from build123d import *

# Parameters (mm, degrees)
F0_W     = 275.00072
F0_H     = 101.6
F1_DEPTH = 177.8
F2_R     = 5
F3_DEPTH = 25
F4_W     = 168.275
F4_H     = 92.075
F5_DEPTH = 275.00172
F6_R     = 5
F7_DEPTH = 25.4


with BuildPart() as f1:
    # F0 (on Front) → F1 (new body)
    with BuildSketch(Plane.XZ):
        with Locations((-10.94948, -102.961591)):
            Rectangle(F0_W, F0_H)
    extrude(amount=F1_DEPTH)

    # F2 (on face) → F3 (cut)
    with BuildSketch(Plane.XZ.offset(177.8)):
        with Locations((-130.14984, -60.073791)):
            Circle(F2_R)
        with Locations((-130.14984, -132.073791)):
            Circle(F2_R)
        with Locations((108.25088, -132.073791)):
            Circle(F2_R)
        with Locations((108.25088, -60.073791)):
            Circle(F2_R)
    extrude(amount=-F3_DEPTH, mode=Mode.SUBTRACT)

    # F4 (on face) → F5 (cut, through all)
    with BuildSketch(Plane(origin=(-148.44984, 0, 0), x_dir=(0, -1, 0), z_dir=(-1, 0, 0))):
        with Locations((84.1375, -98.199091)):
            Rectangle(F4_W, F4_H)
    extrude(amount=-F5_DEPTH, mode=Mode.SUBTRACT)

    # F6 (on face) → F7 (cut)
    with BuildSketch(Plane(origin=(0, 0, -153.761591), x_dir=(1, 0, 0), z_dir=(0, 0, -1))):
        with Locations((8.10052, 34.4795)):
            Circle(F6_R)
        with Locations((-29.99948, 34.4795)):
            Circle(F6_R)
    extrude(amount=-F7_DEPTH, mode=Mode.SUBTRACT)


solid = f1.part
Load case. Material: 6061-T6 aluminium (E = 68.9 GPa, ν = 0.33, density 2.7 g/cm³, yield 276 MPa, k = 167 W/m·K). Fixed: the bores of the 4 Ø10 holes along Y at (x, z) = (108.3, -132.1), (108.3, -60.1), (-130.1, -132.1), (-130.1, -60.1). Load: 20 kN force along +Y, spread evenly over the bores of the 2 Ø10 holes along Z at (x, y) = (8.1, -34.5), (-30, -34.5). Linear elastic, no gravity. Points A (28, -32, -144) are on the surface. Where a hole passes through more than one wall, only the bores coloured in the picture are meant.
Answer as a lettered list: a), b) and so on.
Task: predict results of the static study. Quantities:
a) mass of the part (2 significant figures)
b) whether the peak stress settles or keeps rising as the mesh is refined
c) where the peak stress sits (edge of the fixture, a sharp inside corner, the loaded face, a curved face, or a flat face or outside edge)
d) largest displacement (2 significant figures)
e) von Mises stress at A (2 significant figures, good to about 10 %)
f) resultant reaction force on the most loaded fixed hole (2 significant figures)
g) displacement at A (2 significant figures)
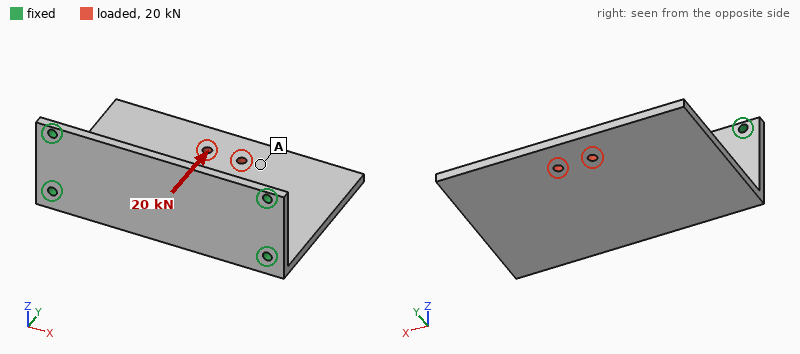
a) 1.9 kg
b) keeps rising
c) edge of the fixture
d) 0.64 mm
e) 14 MPa
f) 12 kN
g) 0.50 mm
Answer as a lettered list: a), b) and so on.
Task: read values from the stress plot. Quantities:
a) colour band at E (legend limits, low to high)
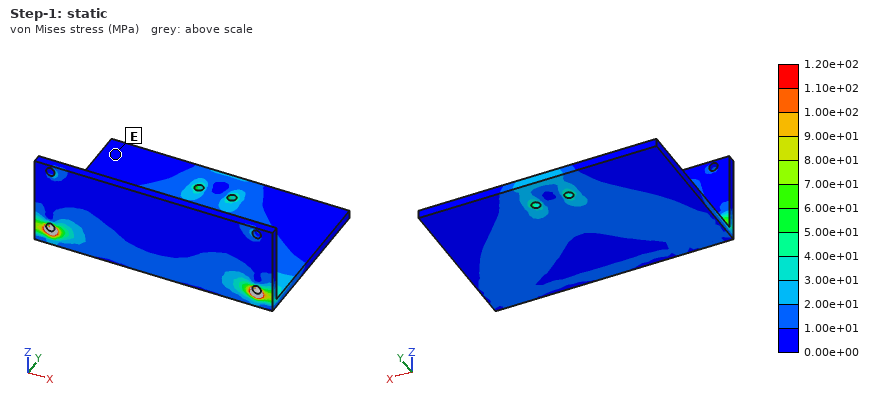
a) 0.00e+00 to 1.00e+01 MPa
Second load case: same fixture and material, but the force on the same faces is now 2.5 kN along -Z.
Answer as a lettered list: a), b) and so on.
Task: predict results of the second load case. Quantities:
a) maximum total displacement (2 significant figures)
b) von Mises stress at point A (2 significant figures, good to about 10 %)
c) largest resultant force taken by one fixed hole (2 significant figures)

a) 3.5 mm
b) 18 MPa
c) 1.7 kN
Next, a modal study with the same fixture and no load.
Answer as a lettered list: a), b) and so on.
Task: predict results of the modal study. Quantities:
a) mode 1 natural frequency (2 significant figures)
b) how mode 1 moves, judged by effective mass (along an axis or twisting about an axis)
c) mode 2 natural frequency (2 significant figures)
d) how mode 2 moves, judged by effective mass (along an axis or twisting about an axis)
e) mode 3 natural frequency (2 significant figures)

a) 210 Hz
b) along Z
c) 420 Hz
d) twisting about Y
e) 970 Hz
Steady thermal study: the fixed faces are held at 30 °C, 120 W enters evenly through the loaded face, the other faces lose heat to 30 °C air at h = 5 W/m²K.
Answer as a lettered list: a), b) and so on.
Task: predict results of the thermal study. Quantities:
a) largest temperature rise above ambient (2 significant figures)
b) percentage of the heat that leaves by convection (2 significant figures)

a) 66 K
b) 16 %
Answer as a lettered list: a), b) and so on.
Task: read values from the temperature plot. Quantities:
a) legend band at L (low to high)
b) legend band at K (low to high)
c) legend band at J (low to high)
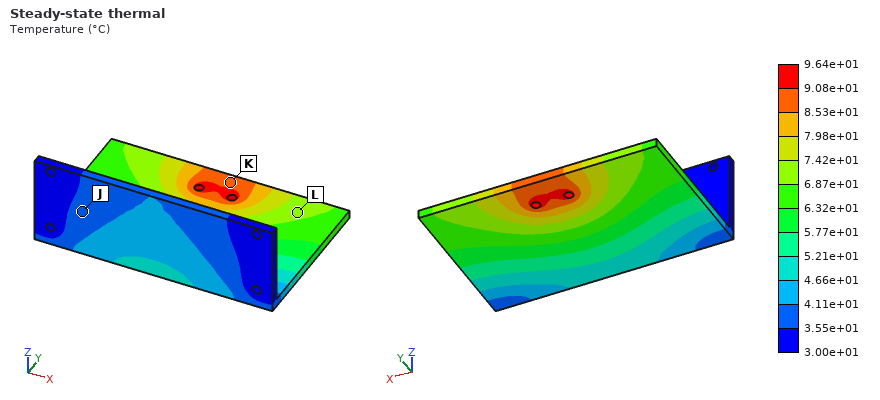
a) 6.87e+01 to 7.42e+01 °C
b) 8.53e+01 to 9.08e+01 °C
c) 3.55e+01 to 4.11e+01 °C
